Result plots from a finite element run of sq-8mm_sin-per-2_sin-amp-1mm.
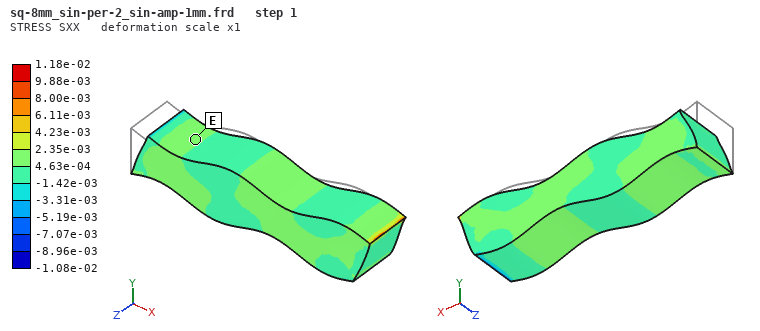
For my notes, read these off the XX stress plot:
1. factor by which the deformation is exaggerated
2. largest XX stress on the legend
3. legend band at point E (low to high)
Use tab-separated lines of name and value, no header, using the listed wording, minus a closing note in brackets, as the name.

factor by which the deformation is exaggerated	1
largest XX stress on the legend	1.18e-02
legend band at point E	4.63e-04 to 2.35e-03
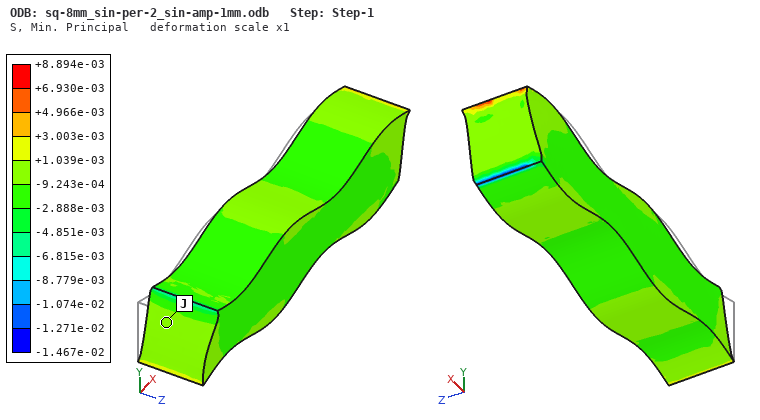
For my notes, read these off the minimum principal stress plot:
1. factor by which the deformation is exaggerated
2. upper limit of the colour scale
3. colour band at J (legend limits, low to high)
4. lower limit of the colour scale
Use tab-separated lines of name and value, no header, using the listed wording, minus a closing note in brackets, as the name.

factor by which the deformation is exaggerated	1
upper limit of the colour scale	+8.894e-03
colour band at J	-9.243e-04 to +1.039e-03
lower limit of the colour scale	-1.467e-02
